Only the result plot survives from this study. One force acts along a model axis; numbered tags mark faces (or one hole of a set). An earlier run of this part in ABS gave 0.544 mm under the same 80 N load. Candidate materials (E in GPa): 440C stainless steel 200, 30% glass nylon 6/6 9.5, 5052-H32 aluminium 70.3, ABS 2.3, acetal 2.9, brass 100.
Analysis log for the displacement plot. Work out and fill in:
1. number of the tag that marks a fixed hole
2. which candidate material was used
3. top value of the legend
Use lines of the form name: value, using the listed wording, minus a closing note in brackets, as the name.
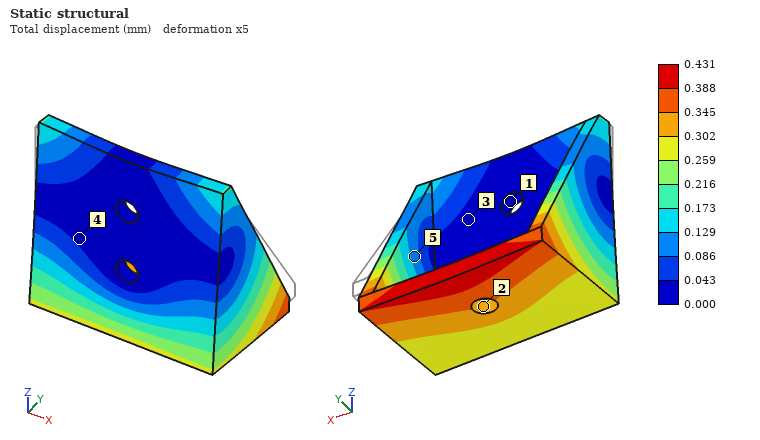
number of the tag that marks a fixed hole: 1
which candidate material was used: acetal
top value of the legend: 0.431 mm
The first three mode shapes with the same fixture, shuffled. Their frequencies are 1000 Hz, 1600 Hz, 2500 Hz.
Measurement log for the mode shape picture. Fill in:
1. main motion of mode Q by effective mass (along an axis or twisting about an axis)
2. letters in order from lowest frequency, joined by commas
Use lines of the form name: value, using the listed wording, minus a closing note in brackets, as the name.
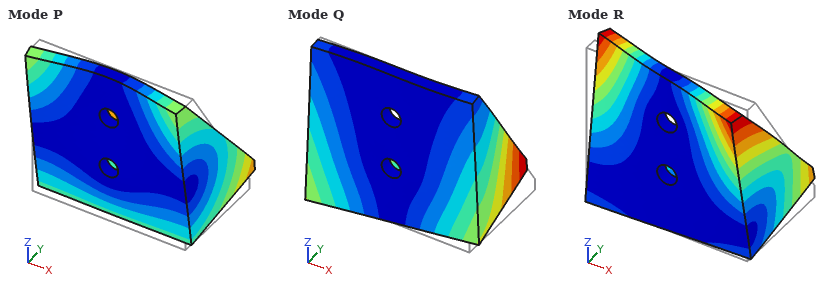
main motion of mode Q by effective mass: along X
letters in order from lowest frequency, joined by commas: Q, P, R
